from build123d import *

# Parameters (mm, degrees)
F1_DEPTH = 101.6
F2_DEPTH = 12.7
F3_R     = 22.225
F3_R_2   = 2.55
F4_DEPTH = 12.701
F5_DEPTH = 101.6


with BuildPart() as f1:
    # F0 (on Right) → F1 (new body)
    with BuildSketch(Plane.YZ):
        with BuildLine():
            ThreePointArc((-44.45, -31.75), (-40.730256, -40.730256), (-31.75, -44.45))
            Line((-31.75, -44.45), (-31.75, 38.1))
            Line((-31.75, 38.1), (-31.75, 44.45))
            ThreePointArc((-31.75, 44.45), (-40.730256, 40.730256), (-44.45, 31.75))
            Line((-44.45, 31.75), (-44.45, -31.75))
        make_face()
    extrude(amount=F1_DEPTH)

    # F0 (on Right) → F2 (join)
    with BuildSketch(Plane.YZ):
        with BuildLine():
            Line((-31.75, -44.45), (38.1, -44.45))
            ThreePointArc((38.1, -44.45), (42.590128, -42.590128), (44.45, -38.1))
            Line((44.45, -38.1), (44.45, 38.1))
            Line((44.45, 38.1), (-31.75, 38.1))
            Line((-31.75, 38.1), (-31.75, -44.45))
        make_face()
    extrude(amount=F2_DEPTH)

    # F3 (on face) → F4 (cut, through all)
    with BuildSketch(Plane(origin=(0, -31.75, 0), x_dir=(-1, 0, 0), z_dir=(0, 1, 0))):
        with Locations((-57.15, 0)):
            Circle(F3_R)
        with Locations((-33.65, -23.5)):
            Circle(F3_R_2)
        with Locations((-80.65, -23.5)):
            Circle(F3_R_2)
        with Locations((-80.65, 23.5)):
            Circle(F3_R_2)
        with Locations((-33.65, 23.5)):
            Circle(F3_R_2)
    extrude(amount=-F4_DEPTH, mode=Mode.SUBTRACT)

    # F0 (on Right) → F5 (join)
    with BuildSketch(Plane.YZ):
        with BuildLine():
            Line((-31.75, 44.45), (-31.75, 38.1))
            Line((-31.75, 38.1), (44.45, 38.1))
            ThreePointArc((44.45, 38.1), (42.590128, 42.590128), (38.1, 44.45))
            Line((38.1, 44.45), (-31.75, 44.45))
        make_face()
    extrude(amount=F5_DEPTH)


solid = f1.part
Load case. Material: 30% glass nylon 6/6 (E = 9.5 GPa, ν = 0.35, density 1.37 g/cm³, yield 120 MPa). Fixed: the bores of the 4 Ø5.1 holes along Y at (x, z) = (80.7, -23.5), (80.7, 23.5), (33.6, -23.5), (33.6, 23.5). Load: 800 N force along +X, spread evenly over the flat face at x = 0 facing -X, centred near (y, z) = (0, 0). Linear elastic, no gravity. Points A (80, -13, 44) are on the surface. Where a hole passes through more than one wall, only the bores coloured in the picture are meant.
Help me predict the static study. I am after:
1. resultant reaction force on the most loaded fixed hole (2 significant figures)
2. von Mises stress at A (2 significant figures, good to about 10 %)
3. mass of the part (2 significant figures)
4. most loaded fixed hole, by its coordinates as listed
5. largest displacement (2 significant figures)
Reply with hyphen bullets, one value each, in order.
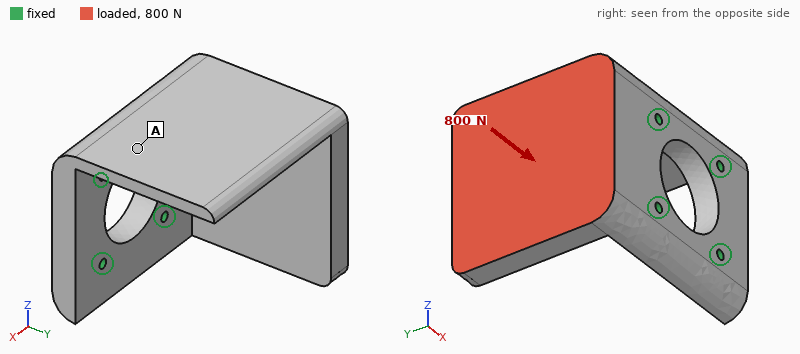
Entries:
- 520 N
- 1.6 MPa
- 290 g
- (33.6, 23.5)
- 0.37 mm
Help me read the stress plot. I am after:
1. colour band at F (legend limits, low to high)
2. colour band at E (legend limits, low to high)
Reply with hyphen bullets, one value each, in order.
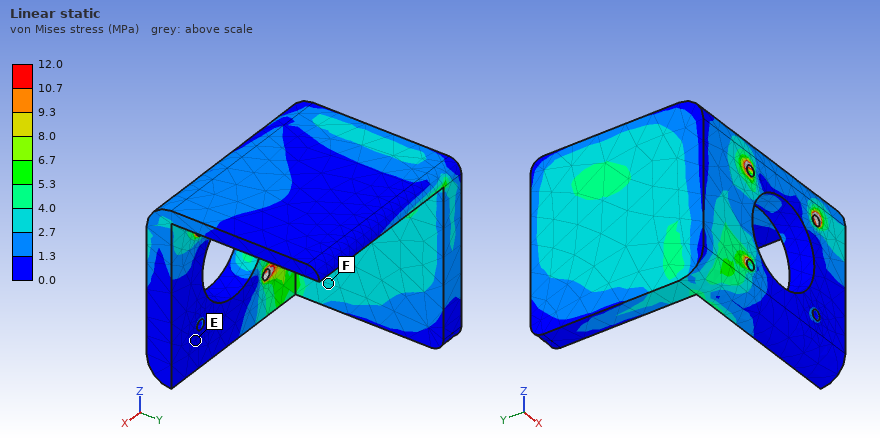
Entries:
- 2.7 to 4.0 MPa
- 0.0 to 1.3 MPa
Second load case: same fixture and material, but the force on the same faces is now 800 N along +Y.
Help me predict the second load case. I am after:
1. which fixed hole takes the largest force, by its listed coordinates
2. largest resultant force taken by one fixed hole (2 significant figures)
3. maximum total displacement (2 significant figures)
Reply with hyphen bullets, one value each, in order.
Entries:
- (33.6, 23.5)
- 670 N
- 0.20 mm
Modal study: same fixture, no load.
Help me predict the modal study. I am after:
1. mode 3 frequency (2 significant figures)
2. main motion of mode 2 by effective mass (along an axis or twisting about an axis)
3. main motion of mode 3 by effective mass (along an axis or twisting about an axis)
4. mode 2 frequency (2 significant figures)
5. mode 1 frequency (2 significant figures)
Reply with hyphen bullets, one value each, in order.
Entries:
- 1100 Hz
- along X
- along Z
- 880 Hz
- 660 Hz
